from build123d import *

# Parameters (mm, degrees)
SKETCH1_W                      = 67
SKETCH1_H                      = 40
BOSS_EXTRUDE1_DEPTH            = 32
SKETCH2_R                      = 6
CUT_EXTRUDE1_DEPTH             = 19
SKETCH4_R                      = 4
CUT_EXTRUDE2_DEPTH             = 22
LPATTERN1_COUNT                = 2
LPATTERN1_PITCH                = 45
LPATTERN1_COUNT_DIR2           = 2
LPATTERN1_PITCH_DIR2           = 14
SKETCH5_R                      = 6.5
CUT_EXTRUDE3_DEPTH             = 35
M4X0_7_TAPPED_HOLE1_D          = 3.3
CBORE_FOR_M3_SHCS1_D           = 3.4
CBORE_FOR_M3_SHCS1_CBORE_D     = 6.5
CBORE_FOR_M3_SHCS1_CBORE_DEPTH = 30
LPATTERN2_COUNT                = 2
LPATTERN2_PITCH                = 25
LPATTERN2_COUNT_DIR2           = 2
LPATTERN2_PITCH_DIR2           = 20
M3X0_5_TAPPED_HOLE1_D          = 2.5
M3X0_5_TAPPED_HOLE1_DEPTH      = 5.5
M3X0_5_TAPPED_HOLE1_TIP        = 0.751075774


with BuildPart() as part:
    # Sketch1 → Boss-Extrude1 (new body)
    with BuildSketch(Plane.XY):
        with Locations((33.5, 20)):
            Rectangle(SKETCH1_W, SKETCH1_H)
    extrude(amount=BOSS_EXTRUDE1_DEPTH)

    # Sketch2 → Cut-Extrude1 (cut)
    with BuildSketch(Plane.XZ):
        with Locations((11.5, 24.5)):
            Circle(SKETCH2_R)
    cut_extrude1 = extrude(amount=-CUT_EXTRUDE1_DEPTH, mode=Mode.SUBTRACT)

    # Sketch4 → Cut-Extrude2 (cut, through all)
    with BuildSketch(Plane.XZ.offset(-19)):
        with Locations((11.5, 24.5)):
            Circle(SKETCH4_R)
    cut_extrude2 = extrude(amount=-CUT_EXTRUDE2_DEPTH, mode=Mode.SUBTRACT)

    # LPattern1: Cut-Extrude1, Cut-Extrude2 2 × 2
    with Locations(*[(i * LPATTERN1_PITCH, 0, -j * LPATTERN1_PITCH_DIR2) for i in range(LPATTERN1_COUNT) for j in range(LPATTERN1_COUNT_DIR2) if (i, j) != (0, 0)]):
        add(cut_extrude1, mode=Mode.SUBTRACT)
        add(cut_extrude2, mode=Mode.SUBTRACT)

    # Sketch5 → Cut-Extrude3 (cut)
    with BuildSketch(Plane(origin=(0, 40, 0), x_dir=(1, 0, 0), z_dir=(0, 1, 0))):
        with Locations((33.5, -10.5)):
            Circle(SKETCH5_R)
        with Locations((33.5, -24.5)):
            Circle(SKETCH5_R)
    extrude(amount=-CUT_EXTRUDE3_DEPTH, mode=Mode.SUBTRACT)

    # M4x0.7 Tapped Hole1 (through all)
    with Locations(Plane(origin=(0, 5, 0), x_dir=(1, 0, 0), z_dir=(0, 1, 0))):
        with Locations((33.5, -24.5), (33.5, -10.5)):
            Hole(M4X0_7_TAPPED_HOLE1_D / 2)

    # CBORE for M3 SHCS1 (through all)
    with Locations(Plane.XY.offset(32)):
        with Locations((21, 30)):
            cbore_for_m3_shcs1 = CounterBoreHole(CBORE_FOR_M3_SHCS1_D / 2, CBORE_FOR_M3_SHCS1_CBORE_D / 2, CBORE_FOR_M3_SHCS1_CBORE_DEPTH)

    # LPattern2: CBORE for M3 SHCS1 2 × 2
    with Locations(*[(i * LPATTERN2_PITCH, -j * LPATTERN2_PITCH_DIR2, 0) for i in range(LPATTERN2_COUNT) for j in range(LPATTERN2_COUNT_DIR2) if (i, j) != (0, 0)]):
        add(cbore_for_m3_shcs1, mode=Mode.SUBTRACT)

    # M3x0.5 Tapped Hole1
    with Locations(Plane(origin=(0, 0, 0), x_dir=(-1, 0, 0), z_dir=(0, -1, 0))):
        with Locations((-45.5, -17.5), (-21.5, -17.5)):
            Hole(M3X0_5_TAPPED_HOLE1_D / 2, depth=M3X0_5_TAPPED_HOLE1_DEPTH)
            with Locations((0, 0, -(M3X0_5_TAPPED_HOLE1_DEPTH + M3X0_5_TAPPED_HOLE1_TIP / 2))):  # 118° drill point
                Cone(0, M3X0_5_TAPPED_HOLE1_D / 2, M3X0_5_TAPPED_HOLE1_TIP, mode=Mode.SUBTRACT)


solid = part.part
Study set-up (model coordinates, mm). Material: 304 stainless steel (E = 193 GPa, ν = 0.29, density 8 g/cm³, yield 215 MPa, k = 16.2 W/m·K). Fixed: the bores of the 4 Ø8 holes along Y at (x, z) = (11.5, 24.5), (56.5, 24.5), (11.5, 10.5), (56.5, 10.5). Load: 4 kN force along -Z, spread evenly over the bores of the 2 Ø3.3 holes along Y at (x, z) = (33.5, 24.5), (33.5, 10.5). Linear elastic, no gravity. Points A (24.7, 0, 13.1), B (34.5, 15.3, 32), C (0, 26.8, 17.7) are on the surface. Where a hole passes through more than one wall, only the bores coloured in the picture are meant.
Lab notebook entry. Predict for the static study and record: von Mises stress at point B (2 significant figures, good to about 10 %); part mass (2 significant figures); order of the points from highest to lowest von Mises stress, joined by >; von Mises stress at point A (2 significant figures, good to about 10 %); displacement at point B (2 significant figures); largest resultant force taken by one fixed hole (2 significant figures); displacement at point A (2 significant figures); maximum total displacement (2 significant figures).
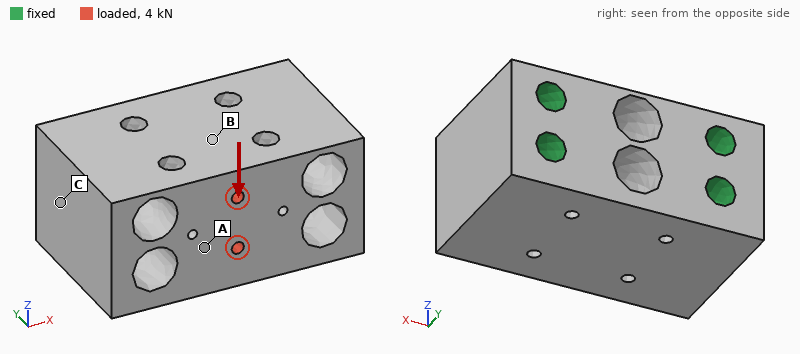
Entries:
7.7 MPa
480 g
A > B > C
15 MPa
2.4 µm
2.2 kN
4.4 µm
6.4 µm
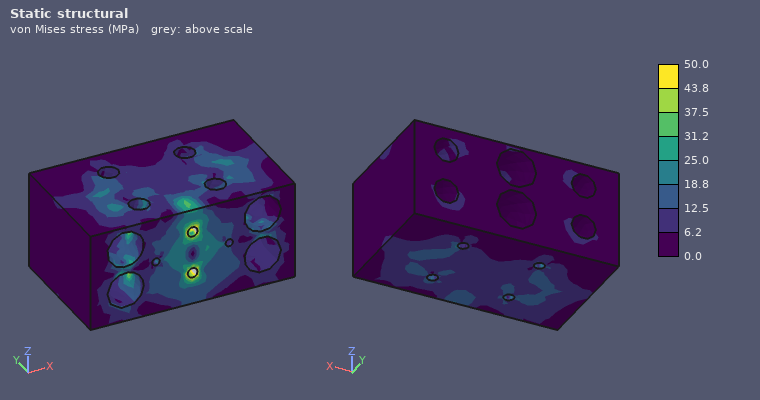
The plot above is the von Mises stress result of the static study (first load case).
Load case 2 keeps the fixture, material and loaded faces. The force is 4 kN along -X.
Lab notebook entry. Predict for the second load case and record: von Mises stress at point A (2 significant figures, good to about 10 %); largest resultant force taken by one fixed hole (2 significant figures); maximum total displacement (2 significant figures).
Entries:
10 MPa
1.5 kN
3.1 µm
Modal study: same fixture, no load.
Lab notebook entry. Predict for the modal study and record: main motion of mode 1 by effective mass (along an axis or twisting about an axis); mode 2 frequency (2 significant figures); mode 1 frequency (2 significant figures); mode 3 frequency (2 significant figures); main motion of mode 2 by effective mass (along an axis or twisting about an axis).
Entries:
along Z
21 kHz
16 kHz
24 kHz
along X
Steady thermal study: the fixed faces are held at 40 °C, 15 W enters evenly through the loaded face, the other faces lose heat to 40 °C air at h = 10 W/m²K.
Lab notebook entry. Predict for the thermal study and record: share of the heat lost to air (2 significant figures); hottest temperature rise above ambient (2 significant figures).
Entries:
11 %
54 K
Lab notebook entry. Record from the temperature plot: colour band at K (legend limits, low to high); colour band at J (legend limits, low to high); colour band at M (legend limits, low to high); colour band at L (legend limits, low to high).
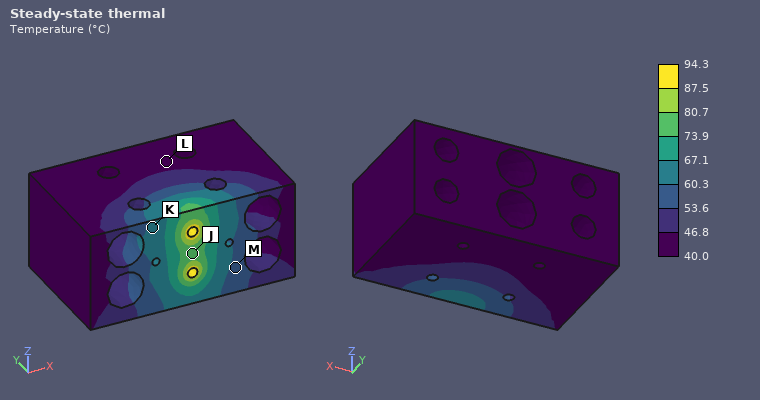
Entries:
60.3 to 67.1 °C
73.9 to 80.7 °C
53.6 to 60.3 °C
40.0 to 46.8 °C
